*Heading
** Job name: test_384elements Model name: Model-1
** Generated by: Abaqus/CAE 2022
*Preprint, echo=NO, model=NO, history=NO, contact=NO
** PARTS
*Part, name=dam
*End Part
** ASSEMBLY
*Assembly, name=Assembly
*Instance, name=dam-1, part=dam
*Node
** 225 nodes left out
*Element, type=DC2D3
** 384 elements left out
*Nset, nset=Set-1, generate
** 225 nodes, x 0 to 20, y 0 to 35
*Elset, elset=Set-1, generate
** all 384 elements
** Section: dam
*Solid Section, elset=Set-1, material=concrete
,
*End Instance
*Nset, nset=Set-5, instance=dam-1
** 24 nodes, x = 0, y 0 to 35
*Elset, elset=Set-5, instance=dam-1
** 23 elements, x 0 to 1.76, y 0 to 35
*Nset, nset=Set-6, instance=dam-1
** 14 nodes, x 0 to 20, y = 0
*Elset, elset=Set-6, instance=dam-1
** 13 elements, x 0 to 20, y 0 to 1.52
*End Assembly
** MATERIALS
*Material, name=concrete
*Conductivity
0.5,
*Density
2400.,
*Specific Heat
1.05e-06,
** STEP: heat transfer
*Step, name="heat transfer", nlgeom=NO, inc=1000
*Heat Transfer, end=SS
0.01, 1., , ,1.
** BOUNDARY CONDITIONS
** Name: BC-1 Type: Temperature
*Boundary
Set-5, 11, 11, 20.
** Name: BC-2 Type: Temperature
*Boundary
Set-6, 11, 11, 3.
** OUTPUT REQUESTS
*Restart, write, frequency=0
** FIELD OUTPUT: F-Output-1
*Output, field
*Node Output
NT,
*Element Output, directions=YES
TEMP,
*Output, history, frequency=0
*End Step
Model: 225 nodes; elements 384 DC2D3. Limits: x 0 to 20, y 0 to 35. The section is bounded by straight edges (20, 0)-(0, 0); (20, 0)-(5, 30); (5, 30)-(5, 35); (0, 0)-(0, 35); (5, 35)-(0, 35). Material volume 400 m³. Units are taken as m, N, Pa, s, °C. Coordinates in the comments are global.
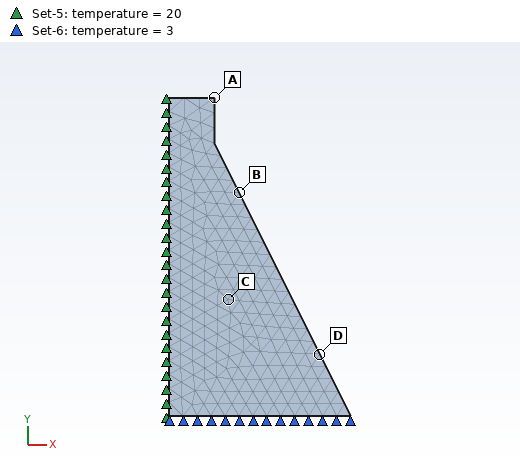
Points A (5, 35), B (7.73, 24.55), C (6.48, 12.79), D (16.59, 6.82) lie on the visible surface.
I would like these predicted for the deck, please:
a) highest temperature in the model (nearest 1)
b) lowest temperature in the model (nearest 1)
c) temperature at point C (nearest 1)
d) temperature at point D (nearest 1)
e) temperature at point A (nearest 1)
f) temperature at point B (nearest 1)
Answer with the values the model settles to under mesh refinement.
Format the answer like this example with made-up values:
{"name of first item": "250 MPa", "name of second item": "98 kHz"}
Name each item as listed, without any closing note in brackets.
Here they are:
{"highest temperature in the model": "20 °C", "lowest temperature in the model": "3 °C", "temperature at point C": "16 °C", "temperature at point D": "7 °C", "temperature at point A": "20 °C", "temperature at point B": "19 °C"}
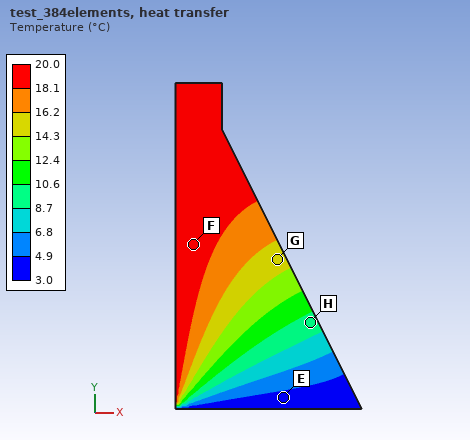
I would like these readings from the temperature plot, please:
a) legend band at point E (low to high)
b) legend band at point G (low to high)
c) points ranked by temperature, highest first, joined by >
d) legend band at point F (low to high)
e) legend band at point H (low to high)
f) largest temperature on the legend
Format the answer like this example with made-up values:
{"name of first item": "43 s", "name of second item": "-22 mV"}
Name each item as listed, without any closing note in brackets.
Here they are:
{"legend band at point E": "3.0 to 4.9 °C", "legend band at point G": "14.3 to 16.2 °C", "points ranked by temperature, highest first, joined by >": "F > G > H > E", "legend band at point F": "18.1 to 20.0 °C", "legend band at point H": "8.7 to 10.6 °C", "largest temperature on the legend": "20.0 °C"}
